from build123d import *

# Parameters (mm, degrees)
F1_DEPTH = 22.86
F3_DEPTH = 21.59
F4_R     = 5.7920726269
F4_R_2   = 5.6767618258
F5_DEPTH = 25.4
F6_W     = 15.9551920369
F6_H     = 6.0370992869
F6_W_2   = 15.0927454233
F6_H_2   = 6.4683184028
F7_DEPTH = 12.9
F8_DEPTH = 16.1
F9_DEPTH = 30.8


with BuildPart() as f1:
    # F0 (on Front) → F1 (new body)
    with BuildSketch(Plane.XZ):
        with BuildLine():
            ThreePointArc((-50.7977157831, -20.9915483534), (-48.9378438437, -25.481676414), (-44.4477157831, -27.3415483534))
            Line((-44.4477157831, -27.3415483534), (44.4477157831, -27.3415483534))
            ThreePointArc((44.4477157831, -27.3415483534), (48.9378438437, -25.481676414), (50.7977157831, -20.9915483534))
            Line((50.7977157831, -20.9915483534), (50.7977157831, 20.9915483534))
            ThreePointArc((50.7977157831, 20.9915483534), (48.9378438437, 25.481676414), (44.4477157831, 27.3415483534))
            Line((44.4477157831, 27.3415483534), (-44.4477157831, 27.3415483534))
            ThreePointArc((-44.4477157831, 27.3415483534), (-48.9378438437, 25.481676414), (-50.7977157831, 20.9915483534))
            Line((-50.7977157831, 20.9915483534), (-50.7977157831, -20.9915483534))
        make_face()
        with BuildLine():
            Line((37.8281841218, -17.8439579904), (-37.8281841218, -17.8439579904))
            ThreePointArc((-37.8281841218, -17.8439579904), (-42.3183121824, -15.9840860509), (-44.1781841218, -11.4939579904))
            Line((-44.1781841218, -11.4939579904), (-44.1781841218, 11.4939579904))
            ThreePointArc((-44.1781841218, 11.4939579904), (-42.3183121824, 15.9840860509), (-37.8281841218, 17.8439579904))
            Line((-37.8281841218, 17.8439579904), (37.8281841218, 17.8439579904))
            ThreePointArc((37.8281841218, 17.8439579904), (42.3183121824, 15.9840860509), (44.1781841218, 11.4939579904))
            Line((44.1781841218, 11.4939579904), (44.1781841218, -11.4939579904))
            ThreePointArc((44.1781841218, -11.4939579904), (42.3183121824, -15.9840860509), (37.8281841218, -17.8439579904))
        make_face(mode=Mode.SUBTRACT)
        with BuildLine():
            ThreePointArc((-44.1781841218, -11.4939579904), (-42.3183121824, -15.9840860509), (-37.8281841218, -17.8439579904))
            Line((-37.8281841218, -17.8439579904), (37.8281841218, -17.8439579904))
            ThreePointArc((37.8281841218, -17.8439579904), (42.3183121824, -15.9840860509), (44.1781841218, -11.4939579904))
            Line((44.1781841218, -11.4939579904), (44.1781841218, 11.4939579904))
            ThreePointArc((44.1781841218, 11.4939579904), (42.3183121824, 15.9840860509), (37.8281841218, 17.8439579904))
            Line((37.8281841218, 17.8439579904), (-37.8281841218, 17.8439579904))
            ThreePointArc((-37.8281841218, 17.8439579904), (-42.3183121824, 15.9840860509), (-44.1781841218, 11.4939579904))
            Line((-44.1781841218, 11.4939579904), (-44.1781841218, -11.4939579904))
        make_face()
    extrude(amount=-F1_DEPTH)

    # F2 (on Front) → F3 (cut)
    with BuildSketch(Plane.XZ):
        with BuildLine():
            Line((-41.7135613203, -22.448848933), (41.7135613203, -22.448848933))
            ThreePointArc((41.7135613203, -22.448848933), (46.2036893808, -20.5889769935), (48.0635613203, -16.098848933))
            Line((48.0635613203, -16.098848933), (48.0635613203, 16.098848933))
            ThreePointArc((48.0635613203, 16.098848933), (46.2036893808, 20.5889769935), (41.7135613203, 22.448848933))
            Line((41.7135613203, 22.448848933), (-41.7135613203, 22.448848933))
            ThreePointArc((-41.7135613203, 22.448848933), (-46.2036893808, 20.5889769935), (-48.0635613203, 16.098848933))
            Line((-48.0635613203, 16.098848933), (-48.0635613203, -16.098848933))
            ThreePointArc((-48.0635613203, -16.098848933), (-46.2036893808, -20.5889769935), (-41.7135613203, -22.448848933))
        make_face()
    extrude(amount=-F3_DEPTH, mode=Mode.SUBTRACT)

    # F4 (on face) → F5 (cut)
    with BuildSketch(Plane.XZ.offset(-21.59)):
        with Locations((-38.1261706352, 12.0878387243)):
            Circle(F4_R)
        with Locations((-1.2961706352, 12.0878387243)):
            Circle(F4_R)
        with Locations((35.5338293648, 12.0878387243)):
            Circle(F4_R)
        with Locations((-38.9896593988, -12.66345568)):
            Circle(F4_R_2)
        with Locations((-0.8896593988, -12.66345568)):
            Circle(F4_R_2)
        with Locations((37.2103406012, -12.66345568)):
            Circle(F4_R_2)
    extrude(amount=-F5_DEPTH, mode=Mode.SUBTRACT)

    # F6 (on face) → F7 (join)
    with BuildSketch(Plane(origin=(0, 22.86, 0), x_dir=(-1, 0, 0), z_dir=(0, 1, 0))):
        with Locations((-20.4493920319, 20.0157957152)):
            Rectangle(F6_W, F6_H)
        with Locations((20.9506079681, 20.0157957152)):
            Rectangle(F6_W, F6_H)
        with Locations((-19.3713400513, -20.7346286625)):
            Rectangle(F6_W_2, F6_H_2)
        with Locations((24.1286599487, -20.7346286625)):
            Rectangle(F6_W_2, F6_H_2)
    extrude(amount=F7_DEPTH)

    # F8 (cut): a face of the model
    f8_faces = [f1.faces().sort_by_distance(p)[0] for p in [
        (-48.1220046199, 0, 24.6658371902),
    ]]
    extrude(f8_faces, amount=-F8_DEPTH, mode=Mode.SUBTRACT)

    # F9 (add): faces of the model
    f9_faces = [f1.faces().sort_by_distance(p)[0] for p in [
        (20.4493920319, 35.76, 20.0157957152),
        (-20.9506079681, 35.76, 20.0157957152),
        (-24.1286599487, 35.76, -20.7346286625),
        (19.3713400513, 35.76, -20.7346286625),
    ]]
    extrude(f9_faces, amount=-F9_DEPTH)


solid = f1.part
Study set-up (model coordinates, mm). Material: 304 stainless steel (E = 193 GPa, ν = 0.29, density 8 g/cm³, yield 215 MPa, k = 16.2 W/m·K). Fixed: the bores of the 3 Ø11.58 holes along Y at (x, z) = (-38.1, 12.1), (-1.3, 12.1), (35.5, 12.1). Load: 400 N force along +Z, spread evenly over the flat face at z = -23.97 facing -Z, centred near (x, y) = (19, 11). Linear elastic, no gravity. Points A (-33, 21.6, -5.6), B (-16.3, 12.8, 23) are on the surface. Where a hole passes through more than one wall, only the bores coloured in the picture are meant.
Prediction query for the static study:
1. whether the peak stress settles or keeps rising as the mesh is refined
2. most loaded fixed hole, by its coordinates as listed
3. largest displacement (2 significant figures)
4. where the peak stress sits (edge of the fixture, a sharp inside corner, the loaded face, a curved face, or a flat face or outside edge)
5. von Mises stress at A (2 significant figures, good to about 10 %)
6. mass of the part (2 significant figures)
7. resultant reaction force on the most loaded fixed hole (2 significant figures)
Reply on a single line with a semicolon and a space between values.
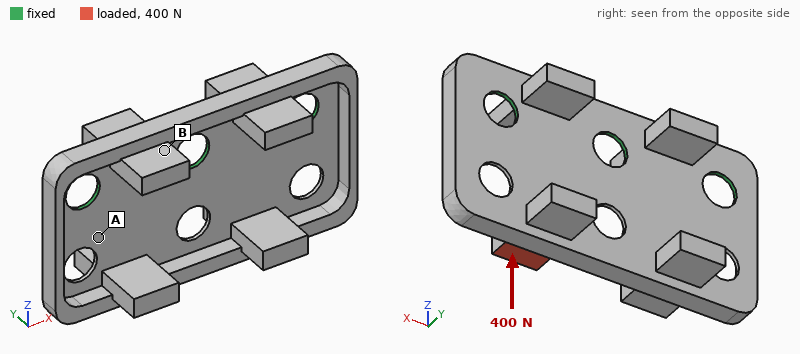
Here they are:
keeps rising; (35.5, 12.1); 0.22 mm; edge of the fixture; 16 MPa; 190 g; 280 N
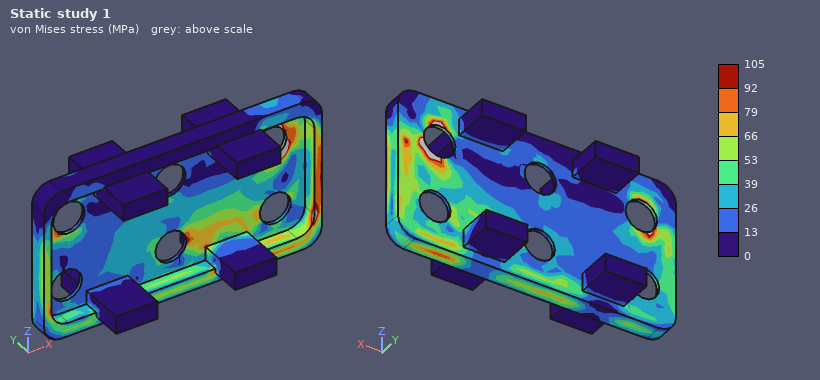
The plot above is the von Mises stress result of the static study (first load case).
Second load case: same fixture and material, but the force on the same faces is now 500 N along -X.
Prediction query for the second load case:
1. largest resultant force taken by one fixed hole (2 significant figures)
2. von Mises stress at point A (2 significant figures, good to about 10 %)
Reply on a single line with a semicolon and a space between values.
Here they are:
330 N; 15 MPa
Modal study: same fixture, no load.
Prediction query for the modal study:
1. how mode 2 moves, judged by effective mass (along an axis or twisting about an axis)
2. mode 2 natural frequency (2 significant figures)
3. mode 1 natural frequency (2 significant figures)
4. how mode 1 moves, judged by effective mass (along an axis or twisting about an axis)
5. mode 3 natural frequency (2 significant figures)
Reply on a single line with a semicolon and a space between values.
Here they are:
twisting about Z; 1300 Hz; 650 Hz; along Y; 2500 Hz
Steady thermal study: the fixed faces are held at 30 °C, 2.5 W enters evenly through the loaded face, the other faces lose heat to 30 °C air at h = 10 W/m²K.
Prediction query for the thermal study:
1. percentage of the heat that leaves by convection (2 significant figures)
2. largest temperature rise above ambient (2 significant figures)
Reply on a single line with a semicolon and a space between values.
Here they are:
59 %; 48 K
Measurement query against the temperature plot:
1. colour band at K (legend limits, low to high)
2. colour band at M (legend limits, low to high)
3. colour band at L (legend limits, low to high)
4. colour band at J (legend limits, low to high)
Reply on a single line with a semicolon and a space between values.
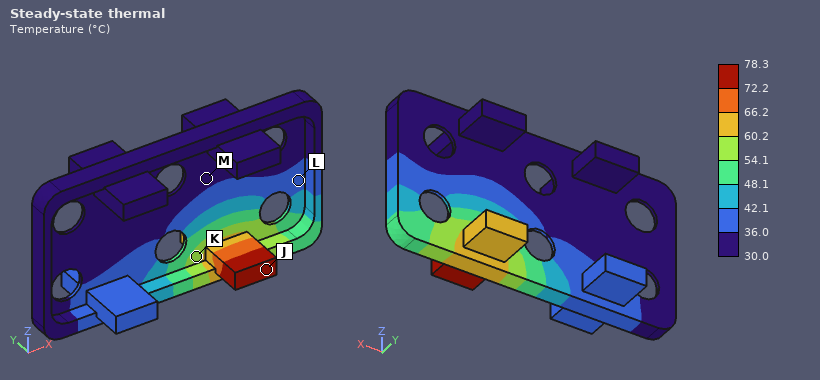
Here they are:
54.1 to 60.2 °C; 30.0 to 36.0 °C; 36.0 to 42.1 °C; 72.2 to 78.3 °C
